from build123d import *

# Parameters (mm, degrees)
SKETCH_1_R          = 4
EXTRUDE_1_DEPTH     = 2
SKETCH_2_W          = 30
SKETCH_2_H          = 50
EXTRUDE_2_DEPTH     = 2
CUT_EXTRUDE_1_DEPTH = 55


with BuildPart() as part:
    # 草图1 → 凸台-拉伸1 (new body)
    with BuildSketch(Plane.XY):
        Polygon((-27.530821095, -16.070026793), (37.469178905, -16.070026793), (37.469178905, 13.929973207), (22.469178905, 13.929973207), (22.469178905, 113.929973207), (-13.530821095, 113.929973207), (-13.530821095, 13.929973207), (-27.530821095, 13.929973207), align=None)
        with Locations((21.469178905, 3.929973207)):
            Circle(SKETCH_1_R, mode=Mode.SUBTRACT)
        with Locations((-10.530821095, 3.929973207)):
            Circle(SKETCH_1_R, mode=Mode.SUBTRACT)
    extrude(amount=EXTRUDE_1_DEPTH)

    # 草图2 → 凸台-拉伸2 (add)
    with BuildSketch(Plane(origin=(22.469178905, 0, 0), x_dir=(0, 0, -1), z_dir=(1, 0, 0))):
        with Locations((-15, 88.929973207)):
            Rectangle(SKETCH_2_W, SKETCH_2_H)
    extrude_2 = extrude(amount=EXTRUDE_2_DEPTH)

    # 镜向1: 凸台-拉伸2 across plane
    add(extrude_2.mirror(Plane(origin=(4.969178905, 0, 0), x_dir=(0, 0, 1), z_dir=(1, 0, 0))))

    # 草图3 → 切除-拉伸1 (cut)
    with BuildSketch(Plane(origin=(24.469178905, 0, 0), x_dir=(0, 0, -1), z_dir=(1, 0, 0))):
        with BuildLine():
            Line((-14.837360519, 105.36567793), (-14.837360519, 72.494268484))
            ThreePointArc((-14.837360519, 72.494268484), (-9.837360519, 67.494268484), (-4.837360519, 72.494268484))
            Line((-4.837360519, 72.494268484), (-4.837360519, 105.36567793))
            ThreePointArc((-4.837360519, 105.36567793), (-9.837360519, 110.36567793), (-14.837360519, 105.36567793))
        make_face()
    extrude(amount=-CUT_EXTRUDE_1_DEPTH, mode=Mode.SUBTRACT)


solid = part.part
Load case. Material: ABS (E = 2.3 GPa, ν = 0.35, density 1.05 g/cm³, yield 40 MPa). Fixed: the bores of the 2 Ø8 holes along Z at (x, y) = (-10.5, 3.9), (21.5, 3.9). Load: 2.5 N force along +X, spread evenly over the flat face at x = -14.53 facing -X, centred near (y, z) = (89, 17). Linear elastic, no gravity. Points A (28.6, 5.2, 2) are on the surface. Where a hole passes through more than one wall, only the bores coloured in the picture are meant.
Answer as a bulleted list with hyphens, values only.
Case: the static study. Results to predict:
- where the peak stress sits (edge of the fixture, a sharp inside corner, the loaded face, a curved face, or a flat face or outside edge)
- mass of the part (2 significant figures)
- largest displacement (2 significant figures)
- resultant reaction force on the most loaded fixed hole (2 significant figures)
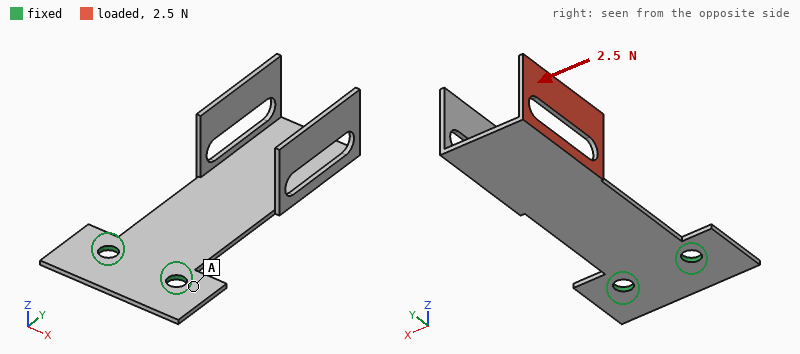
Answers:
- a curved face
- 16 g
- 1.7 mm
- 6.7 N
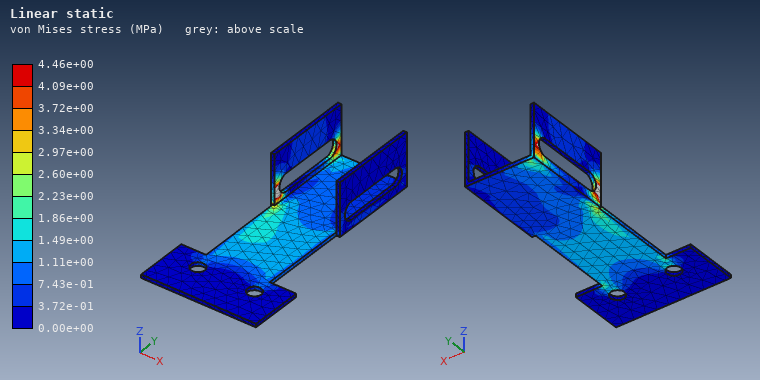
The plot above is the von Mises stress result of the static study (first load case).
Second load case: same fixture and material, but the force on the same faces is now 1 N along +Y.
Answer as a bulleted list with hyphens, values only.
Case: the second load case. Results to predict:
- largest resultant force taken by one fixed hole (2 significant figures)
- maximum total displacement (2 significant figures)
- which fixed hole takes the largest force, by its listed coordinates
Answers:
- 1.1 N
- 1.5 mm
- (-10.5, 3.9)
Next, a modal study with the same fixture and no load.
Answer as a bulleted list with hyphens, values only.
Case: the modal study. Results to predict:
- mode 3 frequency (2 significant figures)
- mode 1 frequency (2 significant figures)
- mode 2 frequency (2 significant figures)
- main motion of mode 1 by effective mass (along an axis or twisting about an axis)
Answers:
- 200 Hz
- 29 Hz
- 96 Hz
- along Z
